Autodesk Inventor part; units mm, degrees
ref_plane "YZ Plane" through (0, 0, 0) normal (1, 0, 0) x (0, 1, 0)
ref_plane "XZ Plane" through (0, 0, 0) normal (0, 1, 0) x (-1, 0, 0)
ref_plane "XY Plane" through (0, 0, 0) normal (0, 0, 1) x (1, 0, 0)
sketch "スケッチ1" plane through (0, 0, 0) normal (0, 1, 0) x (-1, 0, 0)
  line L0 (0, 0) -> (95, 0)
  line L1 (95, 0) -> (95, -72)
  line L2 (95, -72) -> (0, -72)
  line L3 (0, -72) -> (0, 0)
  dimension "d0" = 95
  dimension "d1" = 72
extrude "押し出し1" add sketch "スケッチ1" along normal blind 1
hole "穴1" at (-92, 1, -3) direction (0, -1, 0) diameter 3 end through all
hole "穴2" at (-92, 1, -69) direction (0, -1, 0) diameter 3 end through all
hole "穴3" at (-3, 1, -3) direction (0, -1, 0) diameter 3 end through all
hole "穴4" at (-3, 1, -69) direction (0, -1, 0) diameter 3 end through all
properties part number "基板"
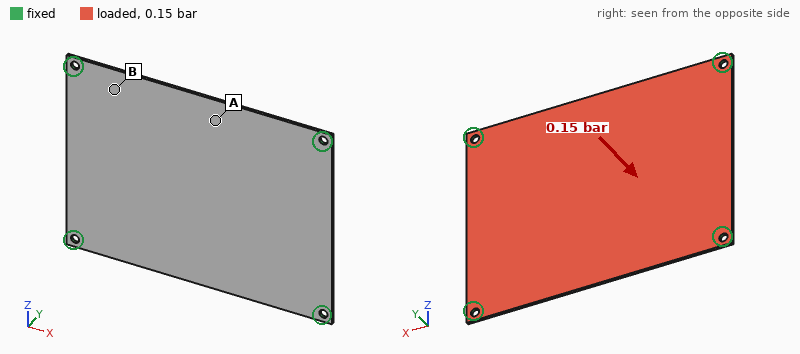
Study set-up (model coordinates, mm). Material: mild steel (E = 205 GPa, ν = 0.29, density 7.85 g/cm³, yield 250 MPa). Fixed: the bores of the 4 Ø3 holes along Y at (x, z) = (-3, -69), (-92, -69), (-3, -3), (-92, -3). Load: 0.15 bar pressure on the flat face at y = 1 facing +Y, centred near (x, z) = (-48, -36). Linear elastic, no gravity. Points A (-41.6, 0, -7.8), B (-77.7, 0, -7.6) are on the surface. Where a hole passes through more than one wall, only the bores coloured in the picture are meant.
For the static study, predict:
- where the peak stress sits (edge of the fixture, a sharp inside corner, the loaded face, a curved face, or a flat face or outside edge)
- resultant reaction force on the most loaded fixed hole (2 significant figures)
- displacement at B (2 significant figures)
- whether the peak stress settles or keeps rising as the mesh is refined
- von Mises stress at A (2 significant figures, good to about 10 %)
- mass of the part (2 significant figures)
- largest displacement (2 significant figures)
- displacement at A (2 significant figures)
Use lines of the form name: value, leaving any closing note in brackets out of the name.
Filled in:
where the peak stress sits: edge of the fixture
resultant reaction force on the most loaded fixed hole: 26 N
displacement at B: 0.086 mm
whether the peak stress settles or keeps rising as the mesh is refined: keeps rising
von Mises stress at A: 39 MPa
mass of the part: 53 g
largest displacement: 0.28 mm
displacement at A: 0.23 mm
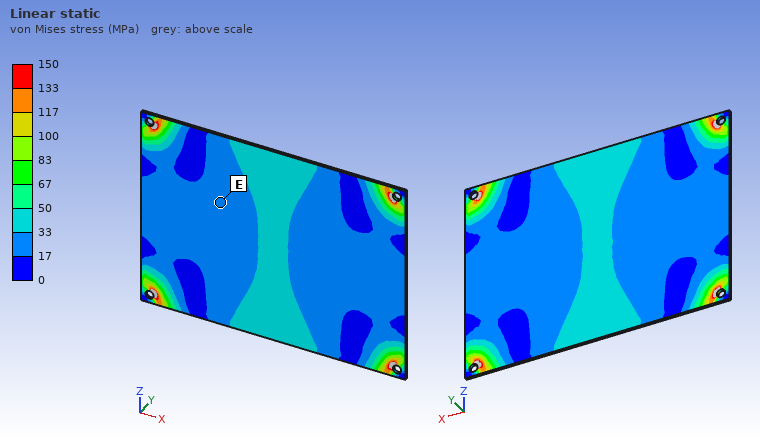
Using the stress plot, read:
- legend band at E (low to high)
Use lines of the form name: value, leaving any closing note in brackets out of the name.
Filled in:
legend band at E: 17 to 33 MPa
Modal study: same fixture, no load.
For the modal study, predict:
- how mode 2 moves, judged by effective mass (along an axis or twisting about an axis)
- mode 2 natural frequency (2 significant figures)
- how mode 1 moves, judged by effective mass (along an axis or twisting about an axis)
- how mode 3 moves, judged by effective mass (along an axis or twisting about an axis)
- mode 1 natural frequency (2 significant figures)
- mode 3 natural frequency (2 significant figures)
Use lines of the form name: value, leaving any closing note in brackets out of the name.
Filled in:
how mode 2 moves, judged by effective mass: twisting about X
mode 2 natural frequency: 840 Hz
how mode 1 moves, judged by effective mass: along Y
how mode 3 moves, judged by effective mass: twisting about Z
mode 1 natural frequency: 490 Hz
mode 3 natural frequency: 1100 Hz
